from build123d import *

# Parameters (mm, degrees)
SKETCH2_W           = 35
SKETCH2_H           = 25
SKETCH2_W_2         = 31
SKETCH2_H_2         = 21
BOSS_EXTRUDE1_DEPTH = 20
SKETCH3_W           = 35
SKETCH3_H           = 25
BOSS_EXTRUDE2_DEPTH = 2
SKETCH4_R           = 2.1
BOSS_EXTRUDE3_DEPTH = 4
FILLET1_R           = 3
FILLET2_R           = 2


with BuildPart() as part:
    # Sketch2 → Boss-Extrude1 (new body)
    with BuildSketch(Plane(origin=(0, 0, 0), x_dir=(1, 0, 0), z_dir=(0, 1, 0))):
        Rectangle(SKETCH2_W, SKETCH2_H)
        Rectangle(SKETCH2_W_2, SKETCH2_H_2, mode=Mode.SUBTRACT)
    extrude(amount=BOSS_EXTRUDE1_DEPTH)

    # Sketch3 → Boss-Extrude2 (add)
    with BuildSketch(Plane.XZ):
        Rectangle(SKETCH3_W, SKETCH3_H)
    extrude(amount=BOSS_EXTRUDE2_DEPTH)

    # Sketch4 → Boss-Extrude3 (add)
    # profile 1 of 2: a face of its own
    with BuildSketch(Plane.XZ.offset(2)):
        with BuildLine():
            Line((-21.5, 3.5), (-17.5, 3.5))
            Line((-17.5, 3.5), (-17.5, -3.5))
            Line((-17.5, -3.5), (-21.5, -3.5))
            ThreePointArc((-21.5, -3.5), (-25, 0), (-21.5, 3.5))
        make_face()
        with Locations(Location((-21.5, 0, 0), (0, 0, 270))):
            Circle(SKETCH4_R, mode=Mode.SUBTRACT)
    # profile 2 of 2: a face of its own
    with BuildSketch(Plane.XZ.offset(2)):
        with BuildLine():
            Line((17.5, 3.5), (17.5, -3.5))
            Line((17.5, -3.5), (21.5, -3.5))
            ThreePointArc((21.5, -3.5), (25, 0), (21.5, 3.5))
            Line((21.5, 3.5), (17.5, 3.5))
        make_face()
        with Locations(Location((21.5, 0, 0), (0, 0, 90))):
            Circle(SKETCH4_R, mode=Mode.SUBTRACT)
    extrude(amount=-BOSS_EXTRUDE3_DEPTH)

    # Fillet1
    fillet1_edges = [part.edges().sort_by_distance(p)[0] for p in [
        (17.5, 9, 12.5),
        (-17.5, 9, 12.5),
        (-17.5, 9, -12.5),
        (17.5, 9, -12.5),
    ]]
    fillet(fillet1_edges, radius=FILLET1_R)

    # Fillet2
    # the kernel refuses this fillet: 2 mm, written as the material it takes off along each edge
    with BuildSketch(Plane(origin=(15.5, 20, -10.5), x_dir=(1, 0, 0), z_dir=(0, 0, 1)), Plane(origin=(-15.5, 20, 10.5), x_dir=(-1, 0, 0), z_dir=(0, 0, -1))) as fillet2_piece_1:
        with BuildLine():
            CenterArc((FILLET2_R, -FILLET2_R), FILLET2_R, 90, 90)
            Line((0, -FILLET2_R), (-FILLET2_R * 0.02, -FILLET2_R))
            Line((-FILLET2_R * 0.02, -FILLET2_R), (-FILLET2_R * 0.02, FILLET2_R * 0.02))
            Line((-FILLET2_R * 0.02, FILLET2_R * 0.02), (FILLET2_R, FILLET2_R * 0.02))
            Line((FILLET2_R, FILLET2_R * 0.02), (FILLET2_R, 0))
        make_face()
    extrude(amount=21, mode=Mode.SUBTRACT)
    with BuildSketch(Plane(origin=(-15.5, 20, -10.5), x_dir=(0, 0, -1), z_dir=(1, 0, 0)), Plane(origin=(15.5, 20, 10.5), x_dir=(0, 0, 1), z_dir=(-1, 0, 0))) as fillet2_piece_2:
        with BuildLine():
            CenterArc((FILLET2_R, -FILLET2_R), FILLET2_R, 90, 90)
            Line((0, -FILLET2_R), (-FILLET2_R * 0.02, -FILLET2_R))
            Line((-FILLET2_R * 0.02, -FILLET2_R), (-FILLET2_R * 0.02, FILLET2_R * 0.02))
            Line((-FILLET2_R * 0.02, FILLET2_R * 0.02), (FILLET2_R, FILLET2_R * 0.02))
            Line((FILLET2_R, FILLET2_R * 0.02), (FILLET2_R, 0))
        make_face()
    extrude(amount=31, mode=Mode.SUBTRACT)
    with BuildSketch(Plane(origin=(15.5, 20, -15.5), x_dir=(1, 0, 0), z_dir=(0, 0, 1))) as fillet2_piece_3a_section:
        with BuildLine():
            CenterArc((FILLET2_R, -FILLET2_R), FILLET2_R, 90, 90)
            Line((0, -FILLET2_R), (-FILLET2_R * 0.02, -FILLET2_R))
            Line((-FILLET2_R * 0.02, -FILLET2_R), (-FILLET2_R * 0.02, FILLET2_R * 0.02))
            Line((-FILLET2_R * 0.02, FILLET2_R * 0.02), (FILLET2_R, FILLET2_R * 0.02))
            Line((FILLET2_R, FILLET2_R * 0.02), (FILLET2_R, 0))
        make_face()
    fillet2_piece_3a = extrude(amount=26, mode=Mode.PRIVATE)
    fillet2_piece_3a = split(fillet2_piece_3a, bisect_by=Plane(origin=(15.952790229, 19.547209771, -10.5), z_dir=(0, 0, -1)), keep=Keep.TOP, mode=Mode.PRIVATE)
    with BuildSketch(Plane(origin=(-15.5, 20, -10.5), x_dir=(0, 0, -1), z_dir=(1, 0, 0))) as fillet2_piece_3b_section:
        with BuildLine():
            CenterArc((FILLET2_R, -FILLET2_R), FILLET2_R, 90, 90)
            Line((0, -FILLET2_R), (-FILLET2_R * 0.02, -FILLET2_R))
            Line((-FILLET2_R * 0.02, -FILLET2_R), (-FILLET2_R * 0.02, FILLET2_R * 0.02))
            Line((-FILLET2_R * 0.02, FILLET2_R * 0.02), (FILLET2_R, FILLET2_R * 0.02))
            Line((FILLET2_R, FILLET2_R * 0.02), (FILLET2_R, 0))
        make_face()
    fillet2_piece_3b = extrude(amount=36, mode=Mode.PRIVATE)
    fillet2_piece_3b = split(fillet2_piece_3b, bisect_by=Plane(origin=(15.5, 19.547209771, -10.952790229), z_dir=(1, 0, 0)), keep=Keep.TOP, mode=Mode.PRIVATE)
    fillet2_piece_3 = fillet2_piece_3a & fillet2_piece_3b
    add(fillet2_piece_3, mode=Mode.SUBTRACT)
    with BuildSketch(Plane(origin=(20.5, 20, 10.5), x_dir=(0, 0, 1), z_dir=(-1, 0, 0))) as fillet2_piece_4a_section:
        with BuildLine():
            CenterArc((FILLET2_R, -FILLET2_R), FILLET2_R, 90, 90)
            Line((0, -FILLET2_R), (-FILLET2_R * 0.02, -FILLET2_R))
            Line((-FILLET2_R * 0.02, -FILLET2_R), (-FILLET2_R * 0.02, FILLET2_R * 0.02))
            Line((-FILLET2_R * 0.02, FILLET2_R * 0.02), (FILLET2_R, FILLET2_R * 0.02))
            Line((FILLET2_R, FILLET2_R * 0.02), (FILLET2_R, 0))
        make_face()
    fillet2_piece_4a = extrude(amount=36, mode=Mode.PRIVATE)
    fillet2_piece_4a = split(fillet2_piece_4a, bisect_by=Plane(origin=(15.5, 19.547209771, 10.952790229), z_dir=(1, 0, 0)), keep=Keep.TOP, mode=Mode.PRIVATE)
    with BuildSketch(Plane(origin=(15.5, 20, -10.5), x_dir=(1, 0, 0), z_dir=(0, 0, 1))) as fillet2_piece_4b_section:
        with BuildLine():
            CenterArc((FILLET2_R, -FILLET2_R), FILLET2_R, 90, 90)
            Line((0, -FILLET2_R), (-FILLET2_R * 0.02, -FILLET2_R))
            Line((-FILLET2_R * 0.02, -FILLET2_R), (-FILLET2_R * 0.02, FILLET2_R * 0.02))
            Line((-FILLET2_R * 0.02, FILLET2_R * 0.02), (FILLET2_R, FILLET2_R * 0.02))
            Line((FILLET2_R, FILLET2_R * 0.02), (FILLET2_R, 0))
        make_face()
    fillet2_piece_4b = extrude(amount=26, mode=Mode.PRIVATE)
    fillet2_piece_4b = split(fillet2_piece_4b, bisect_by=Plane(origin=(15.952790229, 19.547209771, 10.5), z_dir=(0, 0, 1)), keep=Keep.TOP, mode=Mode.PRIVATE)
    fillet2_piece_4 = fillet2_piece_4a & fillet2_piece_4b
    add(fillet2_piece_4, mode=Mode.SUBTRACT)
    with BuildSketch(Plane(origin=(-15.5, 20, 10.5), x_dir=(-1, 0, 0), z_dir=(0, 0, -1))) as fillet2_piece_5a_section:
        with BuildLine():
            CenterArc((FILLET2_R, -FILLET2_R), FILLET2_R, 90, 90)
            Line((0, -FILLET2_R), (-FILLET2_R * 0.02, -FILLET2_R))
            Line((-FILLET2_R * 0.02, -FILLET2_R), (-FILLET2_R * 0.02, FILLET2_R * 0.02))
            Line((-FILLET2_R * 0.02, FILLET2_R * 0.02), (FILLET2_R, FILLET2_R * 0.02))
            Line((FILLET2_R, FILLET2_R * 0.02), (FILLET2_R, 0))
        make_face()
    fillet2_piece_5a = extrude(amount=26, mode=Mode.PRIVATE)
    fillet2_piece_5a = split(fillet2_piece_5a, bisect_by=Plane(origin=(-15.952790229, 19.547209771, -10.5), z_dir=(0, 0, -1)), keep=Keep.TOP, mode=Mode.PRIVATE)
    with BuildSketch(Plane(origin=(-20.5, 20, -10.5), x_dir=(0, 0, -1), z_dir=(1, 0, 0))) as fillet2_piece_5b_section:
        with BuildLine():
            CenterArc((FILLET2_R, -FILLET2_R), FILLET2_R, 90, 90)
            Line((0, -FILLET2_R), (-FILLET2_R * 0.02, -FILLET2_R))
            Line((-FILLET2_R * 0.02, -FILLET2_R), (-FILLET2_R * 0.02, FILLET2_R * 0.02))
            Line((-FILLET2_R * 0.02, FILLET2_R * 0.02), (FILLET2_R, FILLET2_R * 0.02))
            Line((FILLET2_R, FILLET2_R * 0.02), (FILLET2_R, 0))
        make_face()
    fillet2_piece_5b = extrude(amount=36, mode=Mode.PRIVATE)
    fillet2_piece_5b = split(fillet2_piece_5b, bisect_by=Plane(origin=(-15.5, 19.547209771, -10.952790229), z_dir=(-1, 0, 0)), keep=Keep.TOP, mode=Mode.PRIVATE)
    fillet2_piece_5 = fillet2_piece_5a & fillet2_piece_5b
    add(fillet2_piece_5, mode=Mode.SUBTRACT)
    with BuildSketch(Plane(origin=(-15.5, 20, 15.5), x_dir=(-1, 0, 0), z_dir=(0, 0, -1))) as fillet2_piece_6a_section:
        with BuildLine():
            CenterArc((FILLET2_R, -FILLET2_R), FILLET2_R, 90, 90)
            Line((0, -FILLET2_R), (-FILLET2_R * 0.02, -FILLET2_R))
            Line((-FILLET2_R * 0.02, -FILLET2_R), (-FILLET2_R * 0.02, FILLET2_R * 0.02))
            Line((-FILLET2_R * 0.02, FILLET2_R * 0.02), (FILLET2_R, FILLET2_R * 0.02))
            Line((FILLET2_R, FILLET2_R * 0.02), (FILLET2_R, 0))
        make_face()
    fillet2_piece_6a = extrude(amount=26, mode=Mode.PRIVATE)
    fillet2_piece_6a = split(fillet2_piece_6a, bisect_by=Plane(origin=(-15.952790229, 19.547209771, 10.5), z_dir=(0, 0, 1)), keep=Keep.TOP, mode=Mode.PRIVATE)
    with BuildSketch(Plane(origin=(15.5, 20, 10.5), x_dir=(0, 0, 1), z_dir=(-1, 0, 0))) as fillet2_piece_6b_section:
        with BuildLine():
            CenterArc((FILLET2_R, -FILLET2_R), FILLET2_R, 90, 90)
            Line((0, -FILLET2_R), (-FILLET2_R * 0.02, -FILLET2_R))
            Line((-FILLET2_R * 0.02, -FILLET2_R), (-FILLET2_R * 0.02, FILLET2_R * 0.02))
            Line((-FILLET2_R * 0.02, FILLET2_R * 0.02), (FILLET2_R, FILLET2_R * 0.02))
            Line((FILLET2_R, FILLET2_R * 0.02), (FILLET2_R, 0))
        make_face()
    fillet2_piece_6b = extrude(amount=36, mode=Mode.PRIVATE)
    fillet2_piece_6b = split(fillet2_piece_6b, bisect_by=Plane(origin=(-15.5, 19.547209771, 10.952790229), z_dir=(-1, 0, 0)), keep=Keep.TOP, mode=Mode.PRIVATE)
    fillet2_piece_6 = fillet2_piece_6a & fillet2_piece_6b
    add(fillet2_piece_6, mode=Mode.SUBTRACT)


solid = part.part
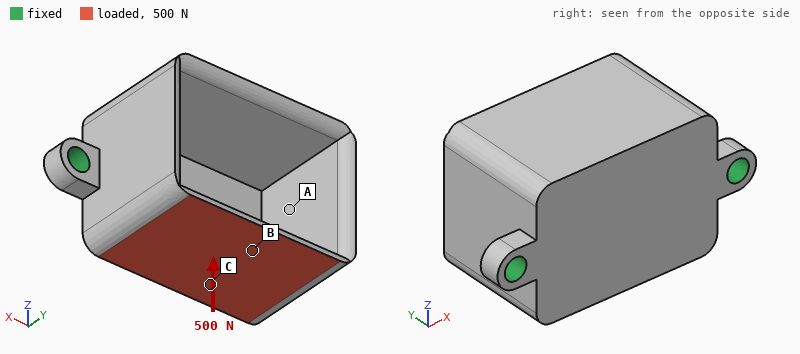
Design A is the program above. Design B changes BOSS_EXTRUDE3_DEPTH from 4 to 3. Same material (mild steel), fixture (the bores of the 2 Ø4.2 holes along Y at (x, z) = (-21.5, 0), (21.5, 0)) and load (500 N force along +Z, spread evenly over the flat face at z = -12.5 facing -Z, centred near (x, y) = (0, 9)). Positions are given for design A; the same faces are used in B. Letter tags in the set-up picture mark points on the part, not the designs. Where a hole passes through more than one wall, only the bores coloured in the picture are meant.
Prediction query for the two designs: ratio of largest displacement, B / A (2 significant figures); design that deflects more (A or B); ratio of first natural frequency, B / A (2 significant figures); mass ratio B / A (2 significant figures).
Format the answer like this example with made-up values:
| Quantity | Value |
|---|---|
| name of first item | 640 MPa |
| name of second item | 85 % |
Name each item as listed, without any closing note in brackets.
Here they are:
| Quantity | Value |
|---|---|
| ratio of largest displacement, B / A | 1.3 |
| design that deflects more | B |
| ratio of first natural frequency, B / A | 0.77 |
| mass ratio B / A | 0.99 |
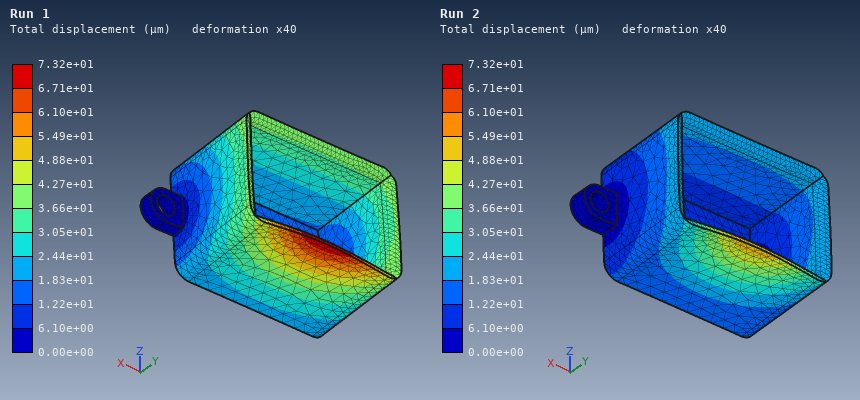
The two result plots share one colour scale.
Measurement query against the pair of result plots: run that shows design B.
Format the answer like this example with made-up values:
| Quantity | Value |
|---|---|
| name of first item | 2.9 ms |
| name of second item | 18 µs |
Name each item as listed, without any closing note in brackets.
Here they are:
| Quantity | Value |
|---|---|
| run that shows design B | Run 1 |
